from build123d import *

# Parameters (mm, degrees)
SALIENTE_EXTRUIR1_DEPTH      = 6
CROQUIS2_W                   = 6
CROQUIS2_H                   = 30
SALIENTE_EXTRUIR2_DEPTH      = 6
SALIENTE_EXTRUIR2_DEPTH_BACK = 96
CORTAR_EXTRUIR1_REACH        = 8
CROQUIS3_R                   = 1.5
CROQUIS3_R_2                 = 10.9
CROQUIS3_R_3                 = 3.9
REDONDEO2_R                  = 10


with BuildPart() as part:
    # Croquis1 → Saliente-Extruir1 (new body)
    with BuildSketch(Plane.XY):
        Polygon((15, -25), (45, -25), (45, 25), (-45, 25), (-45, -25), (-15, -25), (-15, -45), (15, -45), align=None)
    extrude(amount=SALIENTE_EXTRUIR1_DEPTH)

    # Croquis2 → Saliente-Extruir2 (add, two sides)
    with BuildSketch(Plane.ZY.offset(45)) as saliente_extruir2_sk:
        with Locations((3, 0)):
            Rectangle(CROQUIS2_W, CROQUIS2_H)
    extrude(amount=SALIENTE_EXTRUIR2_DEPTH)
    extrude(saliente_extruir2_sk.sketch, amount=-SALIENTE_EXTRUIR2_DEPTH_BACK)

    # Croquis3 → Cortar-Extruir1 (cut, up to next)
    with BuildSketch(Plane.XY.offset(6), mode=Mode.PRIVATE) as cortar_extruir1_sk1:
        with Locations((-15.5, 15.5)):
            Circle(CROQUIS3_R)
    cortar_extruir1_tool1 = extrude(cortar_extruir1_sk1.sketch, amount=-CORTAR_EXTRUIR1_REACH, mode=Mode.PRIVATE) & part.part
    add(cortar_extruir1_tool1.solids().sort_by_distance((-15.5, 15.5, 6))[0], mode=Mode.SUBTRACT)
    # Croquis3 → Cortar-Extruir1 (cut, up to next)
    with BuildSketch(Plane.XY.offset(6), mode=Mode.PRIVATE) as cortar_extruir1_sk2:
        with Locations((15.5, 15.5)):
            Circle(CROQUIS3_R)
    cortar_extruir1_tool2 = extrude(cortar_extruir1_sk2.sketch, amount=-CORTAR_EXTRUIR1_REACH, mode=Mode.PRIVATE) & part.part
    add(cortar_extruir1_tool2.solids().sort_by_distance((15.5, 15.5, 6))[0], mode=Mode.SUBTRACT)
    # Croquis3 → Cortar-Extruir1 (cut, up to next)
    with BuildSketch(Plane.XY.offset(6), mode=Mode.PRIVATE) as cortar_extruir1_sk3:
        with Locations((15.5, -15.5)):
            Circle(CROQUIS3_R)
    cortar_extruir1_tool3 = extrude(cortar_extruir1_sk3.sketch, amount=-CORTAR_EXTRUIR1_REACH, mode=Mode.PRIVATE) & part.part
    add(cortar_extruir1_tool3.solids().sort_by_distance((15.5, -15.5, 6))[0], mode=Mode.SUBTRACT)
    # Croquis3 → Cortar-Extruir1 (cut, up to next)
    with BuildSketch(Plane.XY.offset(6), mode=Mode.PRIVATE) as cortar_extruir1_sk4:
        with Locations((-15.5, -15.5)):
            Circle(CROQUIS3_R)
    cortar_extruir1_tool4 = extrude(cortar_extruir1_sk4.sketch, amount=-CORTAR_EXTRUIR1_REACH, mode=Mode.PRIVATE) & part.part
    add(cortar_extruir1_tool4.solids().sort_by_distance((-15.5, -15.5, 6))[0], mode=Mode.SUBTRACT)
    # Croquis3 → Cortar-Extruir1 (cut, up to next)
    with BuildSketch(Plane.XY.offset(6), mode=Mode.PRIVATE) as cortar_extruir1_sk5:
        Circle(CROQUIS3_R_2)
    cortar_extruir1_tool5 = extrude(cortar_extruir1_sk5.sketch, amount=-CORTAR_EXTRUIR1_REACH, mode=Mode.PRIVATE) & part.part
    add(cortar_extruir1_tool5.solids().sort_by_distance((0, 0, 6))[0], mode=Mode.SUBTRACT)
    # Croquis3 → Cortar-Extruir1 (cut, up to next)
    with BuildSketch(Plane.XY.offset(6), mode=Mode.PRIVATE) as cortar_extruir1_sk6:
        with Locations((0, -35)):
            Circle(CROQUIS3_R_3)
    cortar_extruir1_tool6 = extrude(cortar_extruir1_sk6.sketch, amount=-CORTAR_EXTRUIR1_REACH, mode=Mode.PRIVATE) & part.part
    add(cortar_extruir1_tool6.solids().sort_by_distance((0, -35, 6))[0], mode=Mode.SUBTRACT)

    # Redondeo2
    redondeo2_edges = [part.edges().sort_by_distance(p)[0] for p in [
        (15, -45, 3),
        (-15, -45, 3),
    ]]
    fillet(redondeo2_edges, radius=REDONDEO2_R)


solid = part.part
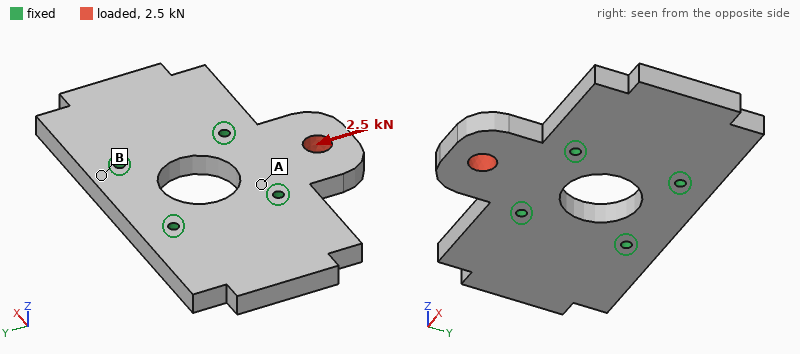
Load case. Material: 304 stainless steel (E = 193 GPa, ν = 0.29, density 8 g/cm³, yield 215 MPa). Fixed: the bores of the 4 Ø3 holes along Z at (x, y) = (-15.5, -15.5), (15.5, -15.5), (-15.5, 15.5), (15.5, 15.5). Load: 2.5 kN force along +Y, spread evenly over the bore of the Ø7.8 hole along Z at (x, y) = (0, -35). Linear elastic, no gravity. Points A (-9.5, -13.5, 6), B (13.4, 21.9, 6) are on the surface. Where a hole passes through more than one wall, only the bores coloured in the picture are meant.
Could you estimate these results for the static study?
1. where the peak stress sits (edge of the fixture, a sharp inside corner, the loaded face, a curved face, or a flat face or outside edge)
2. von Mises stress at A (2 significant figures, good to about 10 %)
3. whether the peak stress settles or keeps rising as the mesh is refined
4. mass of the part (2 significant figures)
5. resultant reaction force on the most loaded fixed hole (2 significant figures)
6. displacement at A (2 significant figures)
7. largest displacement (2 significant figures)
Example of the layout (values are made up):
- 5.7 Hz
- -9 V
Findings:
- edge of the fixture
- 11 MPa
- keeps rising
- 240 g
- 1.2 kN
- 0.72 µm
- 3.4 µm
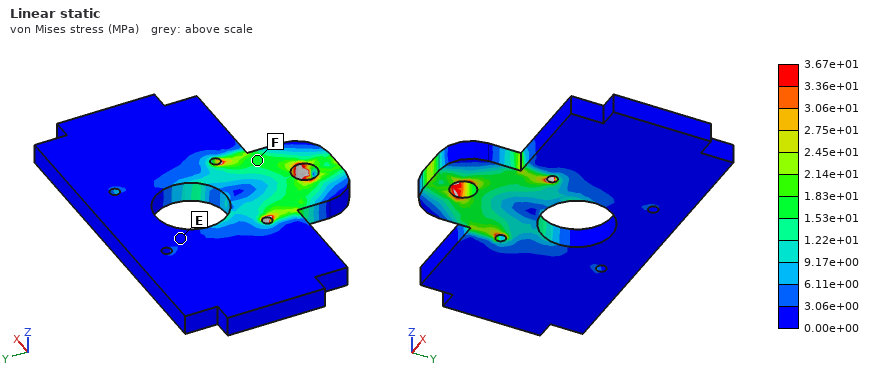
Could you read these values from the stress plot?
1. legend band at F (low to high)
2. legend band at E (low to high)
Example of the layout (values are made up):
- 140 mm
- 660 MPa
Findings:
- 1.53e+01 to 1.83e+01 MPa
- 0.00e+00 to 3.06e+00 MPa
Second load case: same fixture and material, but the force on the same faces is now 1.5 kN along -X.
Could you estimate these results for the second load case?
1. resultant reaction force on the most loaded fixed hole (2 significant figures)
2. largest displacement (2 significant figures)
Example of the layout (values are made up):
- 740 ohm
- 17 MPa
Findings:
- 1.1 kN
- 4.4 µm
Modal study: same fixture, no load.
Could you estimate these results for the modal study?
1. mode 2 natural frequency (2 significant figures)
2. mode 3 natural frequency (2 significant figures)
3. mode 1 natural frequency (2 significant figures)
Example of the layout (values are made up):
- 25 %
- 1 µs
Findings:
- 3700 Hz
- 5600 Hz
- 3600 Hz
